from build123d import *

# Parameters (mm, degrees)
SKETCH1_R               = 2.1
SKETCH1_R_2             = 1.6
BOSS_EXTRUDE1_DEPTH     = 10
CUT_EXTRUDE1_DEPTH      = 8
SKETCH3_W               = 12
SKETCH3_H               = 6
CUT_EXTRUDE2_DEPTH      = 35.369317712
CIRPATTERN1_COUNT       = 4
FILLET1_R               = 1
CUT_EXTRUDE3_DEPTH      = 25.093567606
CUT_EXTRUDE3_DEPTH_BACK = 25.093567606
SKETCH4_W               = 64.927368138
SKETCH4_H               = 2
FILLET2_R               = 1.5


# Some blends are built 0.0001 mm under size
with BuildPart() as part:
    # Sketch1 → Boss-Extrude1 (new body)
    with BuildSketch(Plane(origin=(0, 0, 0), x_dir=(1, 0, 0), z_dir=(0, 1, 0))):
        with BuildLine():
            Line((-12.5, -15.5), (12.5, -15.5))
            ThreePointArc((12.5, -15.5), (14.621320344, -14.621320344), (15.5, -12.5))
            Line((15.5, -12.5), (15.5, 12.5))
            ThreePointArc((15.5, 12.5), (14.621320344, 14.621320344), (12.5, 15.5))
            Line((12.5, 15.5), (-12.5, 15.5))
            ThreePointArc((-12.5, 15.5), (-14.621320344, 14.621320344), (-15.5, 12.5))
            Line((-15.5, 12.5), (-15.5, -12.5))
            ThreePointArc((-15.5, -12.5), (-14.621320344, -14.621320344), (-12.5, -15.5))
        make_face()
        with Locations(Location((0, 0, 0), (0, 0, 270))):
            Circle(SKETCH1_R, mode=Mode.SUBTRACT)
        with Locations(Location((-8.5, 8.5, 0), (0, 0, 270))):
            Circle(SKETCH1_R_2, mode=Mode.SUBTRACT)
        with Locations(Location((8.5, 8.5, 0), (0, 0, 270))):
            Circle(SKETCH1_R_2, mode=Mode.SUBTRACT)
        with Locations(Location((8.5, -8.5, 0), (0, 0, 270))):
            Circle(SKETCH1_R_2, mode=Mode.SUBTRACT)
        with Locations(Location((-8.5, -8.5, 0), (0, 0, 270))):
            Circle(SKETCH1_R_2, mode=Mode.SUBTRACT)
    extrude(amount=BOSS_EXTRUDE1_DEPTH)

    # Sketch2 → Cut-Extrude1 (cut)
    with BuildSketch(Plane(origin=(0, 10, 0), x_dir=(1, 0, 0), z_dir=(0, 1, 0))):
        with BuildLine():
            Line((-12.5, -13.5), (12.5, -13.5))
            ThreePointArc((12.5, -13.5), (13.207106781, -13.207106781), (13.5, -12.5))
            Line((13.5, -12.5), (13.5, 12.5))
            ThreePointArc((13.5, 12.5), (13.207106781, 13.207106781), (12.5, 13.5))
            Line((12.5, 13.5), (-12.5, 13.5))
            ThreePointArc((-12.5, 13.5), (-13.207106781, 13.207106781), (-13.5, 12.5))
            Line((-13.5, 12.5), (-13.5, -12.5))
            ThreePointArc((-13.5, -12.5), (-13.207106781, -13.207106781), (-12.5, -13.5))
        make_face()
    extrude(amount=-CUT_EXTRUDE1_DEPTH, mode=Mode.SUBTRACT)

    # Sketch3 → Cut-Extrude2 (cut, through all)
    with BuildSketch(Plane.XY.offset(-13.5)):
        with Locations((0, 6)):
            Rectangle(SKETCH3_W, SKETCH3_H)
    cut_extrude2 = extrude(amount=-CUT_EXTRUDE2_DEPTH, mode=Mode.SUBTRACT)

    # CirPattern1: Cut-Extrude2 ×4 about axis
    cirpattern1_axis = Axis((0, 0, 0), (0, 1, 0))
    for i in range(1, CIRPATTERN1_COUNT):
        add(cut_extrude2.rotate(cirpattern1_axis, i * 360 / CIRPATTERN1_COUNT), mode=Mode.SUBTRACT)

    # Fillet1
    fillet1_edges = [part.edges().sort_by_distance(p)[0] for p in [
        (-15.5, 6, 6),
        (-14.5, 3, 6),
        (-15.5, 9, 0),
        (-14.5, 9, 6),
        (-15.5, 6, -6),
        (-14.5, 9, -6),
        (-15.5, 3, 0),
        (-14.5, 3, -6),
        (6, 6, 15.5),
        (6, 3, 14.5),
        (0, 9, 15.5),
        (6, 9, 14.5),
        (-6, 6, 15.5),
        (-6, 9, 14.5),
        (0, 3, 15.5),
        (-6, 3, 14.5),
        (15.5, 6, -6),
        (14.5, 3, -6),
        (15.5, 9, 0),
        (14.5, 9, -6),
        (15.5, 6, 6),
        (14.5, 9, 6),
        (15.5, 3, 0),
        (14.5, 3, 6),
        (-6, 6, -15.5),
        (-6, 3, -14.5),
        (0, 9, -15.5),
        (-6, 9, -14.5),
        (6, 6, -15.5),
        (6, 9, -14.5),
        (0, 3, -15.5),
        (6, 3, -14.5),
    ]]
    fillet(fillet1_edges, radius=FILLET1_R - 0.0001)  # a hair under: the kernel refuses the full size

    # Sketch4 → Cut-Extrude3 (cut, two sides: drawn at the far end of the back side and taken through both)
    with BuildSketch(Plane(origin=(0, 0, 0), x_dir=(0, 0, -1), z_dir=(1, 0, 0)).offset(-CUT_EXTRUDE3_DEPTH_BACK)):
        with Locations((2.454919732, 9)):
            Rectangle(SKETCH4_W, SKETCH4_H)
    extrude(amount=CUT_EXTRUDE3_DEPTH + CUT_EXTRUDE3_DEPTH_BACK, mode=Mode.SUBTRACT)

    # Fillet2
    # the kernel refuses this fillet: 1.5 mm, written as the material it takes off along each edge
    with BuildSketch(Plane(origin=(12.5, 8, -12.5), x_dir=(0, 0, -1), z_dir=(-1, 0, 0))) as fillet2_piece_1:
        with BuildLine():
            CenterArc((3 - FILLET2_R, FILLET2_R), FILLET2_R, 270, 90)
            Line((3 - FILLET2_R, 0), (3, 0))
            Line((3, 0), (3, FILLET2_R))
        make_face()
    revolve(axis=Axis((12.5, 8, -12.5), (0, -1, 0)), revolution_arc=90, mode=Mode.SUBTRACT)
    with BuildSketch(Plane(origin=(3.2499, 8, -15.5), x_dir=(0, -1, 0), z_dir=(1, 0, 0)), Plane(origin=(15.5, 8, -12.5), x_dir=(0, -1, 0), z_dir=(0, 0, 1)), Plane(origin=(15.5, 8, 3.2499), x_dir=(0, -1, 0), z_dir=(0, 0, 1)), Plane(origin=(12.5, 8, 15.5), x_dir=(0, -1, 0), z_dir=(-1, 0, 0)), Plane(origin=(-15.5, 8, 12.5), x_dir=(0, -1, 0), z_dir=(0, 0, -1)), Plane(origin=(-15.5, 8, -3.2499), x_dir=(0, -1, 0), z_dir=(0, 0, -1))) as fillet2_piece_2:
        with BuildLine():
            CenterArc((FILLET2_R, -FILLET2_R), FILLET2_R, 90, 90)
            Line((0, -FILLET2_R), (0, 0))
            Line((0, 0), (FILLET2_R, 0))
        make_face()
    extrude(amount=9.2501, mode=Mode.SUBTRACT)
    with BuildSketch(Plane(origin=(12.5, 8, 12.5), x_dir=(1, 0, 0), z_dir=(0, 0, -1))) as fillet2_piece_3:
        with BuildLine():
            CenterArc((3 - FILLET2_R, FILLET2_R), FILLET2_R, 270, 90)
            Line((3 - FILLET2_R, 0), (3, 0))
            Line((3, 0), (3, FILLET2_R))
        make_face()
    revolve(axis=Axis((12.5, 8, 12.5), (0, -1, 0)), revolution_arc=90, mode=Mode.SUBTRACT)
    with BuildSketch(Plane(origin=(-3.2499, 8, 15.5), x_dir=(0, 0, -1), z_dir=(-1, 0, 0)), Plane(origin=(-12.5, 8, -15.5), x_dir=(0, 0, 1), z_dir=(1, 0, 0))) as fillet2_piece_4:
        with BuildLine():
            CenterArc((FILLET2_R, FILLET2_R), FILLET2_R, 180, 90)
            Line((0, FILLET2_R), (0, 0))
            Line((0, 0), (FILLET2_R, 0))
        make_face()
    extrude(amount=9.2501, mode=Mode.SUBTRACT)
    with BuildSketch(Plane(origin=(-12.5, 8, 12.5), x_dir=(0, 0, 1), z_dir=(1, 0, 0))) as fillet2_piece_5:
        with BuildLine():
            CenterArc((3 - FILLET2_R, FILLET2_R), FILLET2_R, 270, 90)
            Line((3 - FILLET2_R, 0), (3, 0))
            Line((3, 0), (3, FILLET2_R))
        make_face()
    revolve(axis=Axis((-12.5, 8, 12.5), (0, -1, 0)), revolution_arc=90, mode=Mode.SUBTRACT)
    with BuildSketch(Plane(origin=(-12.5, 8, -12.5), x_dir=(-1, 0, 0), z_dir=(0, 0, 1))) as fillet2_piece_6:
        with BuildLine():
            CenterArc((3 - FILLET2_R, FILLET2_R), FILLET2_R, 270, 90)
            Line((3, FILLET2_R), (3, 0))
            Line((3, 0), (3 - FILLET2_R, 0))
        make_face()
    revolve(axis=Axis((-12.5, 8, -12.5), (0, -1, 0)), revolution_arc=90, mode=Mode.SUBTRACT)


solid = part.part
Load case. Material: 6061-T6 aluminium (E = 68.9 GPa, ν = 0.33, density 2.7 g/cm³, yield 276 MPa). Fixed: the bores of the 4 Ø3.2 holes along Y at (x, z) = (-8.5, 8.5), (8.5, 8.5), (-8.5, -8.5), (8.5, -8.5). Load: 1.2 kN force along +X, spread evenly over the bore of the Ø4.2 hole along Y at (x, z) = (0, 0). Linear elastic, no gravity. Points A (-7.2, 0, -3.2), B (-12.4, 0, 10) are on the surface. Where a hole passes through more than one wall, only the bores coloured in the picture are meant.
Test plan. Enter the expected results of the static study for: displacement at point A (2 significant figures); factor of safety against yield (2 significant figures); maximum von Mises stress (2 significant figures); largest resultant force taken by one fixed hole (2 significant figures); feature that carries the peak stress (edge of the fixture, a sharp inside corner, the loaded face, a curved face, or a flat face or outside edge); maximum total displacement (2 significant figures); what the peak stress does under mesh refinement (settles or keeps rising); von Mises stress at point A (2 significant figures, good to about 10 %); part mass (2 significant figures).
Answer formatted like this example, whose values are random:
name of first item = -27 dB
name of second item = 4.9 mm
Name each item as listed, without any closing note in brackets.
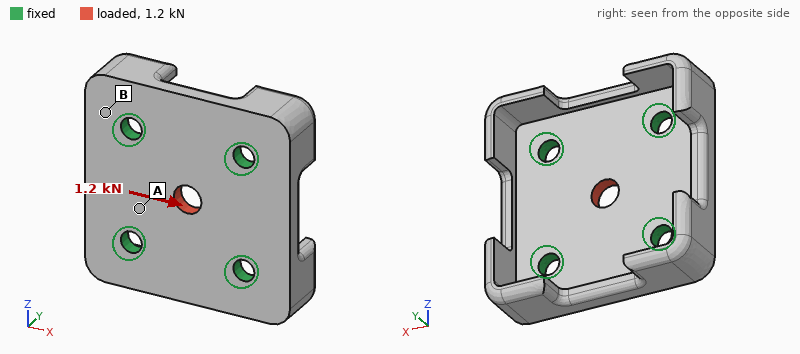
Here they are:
displacement at point A = 2.0 µm
factor of safety against yield = 3.5
maximum von Mises stress = 80 MPa
largest resultant force taken by one fixed hole = 320 N
feature that carries the peak stress = the loaded face
maximum total displacement = 4.8 µm
what the peak stress does under mesh refinement = settles
von Mises stress at point A = 18 MPa
part mass = 7.1 g
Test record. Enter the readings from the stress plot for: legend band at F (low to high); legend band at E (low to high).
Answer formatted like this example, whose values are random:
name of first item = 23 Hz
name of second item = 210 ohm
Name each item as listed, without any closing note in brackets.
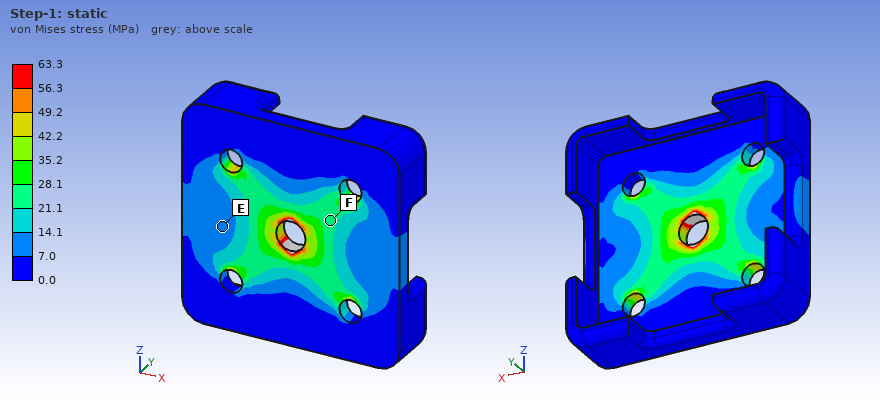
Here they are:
legend band at F = 21.1 to 28.1 MPa
legend band at E = 7.0 to 14.1 MPa
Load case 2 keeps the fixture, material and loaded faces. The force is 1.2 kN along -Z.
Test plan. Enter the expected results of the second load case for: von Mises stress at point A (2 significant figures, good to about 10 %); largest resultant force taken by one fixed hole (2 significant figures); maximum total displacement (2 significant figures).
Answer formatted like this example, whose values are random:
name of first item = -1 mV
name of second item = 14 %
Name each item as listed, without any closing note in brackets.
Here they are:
von Mises stress at point A = 14 MPa
largest resultant force taken by one fixed hole = 320 N
maximum total displacement = 4.8 µm
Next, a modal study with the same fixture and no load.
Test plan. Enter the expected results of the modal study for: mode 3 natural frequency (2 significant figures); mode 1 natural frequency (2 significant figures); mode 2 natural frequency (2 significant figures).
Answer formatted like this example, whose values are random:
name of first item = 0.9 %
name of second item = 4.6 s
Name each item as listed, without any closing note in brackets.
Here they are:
mode 3 natural frequency = 18 kHz
mode 1 natural frequency = 18 kHz
mode 2 natural frequency = 18 kHz
